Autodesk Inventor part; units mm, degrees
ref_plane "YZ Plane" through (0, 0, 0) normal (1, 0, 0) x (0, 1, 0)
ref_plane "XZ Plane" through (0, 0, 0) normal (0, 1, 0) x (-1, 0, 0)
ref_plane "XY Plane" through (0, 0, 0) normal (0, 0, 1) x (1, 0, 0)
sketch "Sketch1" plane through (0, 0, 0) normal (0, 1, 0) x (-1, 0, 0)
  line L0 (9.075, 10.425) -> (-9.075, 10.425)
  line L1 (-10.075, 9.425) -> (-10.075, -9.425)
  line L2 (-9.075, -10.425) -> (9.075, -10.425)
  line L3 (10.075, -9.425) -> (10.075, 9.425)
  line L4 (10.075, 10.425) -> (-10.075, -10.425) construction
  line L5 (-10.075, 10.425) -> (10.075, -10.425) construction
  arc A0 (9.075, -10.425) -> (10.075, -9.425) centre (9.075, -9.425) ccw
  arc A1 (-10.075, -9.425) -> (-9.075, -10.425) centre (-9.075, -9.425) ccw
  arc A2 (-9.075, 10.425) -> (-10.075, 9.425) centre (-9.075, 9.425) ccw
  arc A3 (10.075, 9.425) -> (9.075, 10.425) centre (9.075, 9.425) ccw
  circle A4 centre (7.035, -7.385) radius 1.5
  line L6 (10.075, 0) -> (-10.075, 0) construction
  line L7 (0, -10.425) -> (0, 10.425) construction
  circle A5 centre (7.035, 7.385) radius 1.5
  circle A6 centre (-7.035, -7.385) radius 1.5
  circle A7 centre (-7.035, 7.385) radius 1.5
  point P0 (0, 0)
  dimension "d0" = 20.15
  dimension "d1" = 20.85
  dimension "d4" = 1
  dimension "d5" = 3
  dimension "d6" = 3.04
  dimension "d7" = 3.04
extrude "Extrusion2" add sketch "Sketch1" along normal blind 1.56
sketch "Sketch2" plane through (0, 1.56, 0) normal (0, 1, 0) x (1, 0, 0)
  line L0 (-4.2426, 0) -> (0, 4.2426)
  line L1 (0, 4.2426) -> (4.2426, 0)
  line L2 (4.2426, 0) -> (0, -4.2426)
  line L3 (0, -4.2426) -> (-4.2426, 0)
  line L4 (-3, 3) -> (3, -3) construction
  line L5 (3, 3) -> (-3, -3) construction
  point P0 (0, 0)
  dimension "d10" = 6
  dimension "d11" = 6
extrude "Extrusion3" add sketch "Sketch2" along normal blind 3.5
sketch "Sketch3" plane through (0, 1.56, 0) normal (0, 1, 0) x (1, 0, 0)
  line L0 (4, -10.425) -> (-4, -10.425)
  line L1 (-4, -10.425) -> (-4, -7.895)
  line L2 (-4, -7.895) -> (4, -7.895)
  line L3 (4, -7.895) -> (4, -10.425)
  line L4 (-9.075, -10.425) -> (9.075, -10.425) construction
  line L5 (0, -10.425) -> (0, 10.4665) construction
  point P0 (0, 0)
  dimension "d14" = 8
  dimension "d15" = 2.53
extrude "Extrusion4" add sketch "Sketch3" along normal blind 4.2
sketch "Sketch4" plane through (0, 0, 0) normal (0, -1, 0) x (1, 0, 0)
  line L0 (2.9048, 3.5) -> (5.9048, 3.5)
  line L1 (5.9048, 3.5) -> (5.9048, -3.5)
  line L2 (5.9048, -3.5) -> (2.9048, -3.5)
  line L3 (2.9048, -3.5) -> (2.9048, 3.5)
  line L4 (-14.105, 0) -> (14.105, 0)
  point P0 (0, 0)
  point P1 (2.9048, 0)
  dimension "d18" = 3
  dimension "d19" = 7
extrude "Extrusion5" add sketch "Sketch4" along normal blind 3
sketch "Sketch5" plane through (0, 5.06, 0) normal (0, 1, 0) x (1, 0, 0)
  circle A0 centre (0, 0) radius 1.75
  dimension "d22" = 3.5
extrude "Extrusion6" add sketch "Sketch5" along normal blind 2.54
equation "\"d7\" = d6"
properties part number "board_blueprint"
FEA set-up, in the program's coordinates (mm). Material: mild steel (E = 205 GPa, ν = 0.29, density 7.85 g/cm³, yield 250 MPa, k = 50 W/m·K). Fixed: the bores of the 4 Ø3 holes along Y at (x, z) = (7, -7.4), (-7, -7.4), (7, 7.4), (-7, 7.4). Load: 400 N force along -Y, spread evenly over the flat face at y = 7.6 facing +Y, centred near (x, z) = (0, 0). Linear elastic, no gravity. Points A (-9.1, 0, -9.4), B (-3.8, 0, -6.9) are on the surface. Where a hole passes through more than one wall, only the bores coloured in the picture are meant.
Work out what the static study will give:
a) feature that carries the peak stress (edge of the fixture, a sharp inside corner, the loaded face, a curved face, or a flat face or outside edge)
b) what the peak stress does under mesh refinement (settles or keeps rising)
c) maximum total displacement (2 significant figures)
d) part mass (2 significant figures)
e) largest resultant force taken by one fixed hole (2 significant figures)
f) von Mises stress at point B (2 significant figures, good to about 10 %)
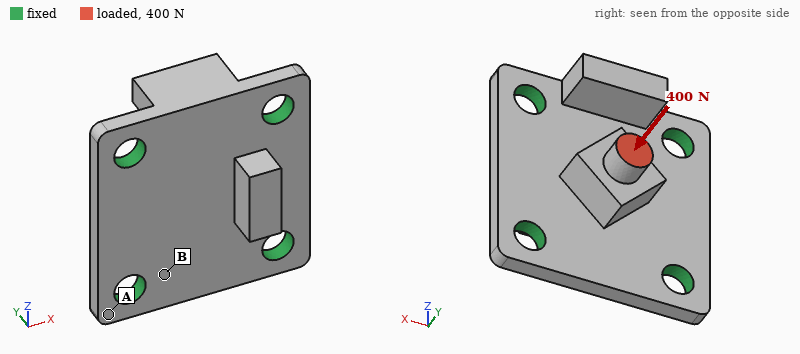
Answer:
edge of the fixture
keeps rising
6.0 µm
7.1 g
100 N
36 MPa
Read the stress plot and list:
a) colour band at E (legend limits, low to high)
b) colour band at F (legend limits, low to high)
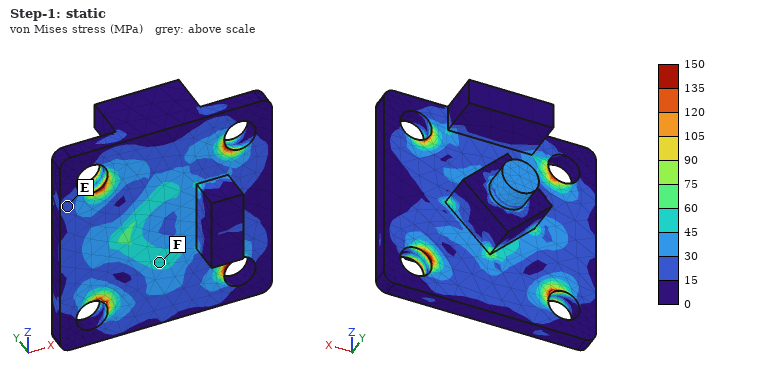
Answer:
15 to 30 MPa
45 to 60 MPa
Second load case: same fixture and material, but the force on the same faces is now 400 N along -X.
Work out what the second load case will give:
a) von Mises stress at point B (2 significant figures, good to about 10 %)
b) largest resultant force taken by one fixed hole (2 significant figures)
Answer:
32 MPa
170 N
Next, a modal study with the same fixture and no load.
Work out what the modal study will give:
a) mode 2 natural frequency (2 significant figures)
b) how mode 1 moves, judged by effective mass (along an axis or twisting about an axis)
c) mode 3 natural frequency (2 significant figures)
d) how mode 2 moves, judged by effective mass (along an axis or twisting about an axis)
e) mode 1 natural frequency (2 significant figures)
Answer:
34 kHz
along Y
39 kHz
along Y
27 kHz
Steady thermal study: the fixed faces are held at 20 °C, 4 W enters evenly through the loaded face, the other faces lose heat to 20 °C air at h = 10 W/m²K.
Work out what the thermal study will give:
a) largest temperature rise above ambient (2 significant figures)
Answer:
45 K
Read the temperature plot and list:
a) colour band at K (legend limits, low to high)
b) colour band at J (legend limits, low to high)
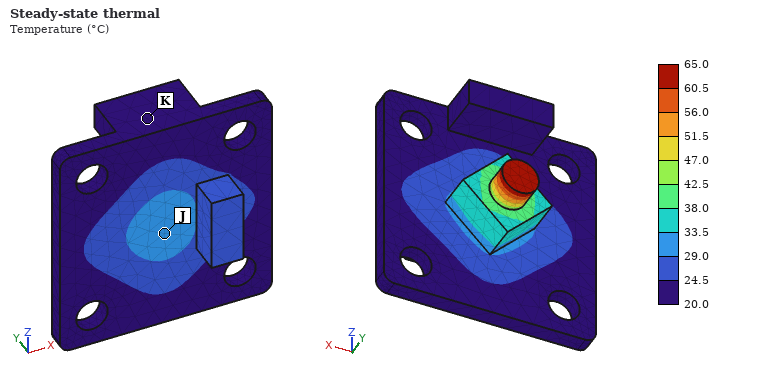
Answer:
20.0 to 24.5 °C
29.0 to 33.5 °C
